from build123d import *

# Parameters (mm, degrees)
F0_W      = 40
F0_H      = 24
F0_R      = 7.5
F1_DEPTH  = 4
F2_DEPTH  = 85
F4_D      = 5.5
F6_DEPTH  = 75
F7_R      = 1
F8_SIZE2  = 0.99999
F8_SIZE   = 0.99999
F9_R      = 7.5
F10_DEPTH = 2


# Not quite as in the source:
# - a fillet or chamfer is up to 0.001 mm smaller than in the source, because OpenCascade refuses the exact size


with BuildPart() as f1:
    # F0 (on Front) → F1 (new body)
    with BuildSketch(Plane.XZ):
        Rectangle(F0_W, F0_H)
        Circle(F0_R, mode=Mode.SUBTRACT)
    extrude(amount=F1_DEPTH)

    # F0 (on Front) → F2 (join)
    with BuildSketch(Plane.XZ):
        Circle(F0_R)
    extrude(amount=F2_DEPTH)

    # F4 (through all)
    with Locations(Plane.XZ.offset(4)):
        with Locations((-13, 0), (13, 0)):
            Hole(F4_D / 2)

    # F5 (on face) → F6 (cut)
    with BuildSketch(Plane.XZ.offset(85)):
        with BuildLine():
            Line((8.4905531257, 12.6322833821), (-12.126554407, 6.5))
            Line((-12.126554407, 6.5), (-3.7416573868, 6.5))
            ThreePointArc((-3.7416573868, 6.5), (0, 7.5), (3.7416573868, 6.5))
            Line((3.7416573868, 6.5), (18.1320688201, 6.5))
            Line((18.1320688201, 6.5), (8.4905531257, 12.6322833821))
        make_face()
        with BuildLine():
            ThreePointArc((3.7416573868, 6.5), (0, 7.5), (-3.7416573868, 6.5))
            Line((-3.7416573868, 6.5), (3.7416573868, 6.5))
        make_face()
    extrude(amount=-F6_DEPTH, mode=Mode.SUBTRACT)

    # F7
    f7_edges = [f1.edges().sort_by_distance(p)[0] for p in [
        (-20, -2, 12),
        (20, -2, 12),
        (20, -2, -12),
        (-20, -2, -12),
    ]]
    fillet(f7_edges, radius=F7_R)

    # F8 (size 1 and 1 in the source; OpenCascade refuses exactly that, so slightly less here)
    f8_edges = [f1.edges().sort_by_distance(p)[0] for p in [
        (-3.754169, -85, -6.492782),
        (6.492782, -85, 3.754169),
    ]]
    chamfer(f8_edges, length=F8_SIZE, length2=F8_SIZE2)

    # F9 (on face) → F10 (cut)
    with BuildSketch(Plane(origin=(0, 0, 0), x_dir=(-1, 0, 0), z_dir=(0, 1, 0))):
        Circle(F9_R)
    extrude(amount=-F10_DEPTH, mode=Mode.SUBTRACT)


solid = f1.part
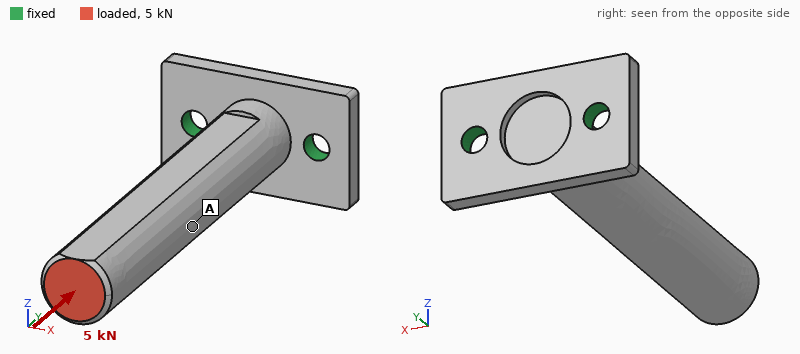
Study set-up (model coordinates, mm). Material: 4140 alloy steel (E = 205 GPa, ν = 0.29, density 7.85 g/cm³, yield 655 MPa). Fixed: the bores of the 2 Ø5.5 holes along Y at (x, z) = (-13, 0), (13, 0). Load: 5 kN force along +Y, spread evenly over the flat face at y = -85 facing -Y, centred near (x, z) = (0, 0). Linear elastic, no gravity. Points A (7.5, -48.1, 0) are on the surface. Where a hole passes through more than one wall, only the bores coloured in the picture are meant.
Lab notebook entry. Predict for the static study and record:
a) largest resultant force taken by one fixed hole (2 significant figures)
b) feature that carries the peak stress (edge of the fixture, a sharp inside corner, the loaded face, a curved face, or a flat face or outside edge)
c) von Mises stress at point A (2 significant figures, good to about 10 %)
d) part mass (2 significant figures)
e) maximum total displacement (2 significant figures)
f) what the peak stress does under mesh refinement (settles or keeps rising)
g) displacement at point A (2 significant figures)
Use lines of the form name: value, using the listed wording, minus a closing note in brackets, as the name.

largest resultant force taken by one fixed hole: 2.8 kN
feature that carries the peak stress: edge of the fixture
von Mises stress at point A: 29 MPa
part mass: 140 g
maximum total displacement: 22 µm
what the peak stress does under mesh refinement: keeps rising
displacement at point A: 15 µm
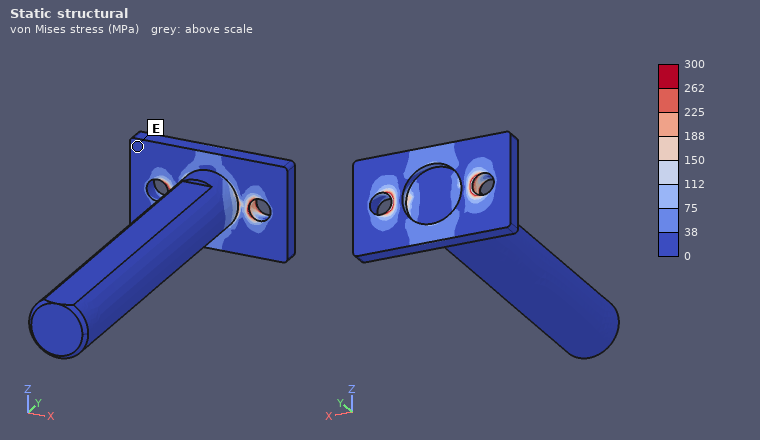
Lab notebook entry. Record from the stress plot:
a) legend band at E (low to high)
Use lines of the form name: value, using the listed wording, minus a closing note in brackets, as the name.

legend band at E: 0 to 38 MPa
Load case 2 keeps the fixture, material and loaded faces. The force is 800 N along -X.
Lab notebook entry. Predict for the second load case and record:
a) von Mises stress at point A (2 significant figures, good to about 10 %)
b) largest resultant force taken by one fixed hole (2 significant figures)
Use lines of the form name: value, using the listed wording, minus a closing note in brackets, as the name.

von Mises stress at point A: 90 MPa
largest resultant force taken by one fixed hole: 3.8 kN
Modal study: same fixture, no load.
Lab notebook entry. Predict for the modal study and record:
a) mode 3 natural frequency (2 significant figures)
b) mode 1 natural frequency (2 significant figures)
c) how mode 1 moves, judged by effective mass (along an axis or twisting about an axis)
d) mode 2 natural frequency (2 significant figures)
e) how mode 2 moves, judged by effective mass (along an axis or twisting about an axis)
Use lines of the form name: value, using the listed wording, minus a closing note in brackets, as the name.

mode 3 natural frequency: 6700 Hz
mode 1 natural frequency: 840 Hz
how mode 1 moves, judged by effective mass: along Z
mode 2 natural frequency: 1300 Hz
how mode 2 moves, judged by effective mass: along X
